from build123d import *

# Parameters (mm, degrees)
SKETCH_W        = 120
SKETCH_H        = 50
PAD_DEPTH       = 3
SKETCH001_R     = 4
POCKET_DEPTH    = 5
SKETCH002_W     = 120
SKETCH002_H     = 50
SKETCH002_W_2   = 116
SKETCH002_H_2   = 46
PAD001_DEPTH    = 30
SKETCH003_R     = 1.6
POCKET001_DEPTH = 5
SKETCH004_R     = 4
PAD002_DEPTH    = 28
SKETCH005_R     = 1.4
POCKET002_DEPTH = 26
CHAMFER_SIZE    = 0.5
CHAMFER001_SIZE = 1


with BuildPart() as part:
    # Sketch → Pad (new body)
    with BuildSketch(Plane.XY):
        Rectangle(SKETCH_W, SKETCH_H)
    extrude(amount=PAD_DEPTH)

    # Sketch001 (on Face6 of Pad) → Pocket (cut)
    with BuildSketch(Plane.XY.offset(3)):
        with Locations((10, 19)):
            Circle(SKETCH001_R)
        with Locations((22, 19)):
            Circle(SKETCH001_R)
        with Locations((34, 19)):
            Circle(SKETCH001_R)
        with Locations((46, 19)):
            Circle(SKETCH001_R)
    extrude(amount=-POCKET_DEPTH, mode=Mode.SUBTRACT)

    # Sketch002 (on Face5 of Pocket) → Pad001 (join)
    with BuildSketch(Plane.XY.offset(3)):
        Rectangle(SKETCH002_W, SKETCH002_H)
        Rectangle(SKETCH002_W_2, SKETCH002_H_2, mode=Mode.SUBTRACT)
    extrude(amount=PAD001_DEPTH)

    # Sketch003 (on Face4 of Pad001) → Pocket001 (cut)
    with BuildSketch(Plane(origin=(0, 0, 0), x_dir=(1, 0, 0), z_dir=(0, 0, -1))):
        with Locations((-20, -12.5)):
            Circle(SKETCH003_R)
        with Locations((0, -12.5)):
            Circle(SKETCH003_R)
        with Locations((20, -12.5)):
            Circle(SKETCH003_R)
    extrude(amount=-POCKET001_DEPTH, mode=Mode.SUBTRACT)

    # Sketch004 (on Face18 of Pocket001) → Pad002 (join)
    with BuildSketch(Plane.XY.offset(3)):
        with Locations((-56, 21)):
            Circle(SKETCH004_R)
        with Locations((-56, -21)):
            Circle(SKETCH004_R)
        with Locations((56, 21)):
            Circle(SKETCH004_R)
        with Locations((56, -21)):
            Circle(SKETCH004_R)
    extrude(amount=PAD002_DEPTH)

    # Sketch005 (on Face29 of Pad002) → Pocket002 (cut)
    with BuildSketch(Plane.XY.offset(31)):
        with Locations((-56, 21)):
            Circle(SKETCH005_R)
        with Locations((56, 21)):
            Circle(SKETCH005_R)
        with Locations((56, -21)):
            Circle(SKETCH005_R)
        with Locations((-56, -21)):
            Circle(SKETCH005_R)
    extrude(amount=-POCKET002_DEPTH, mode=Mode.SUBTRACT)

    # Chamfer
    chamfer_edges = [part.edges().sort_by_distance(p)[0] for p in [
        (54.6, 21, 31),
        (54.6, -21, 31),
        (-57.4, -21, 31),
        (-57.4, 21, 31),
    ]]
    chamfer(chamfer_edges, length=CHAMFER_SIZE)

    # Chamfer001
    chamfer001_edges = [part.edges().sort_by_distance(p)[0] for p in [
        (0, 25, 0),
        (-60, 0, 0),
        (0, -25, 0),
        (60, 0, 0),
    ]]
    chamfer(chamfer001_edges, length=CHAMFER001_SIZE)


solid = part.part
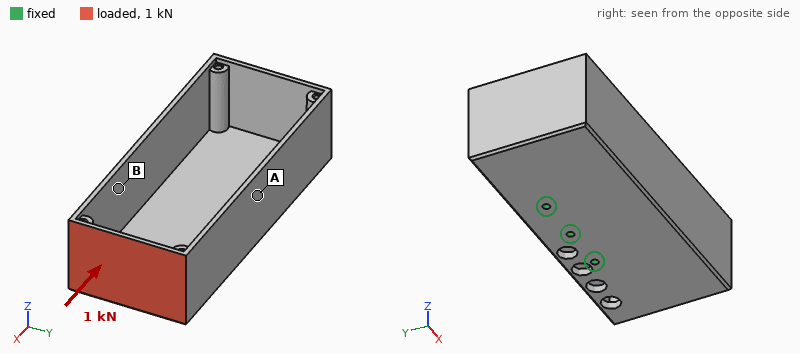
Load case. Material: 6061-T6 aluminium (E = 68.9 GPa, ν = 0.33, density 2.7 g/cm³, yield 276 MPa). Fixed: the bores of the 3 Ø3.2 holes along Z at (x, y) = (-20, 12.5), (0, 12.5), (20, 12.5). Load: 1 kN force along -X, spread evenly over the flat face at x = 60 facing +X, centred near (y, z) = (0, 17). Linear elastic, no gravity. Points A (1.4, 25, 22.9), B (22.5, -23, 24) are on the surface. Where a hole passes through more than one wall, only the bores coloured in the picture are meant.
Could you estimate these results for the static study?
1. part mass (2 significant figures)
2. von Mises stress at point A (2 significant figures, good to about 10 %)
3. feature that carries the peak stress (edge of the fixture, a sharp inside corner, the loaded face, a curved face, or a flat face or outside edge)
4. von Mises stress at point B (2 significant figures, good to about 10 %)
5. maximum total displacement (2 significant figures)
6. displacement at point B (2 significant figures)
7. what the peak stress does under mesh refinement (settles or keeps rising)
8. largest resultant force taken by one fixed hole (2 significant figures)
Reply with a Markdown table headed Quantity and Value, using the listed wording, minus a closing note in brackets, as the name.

| Quantity | Value |
|---|---|
| part mass | 110 g |
| von Mises stress at point A | 16 MPa |
| feature that carries the peak stress | edge of the fixture |
| von Mises stress at point B | 6.7 MPa |
| maximum total displacement | 0.30 mm |
| displacement at point B | 0.13 mm |
| what the peak stress does under mesh refinement | keeps rising |
| largest resultant force taken by one fixed hole | 560 N |
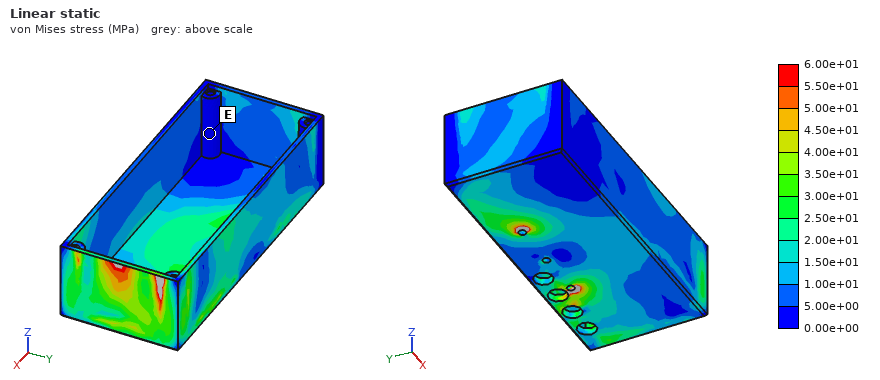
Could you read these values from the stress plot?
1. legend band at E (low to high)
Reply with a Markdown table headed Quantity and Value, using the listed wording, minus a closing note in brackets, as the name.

| Quantity | Value |
|---|---|
| legend band at E | 0.00e+00 to 5.00e+00 MPa |
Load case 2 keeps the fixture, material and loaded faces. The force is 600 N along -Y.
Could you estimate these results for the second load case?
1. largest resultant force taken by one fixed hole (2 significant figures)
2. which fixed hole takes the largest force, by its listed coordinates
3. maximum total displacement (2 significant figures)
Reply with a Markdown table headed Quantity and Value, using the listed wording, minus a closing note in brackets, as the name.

| Quantity | Value |
|---|---|
| largest resultant force taken by one fixed hole | 1.2 kN |
| which fixed hole takes the largest force, by its listed coordinates | (20, 12.5) |
| maximum total displacement | 0.81 mm |
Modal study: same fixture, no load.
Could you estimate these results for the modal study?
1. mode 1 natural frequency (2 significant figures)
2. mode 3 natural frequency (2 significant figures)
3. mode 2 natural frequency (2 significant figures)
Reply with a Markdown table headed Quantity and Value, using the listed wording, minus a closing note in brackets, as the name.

| Quantity | Value |
|---|---|
| mode 1 natural frequency | 670 Hz |
| mode 3 natural frequency | 1400 Hz |
| mode 2 natural frequency | 720 Hz |
